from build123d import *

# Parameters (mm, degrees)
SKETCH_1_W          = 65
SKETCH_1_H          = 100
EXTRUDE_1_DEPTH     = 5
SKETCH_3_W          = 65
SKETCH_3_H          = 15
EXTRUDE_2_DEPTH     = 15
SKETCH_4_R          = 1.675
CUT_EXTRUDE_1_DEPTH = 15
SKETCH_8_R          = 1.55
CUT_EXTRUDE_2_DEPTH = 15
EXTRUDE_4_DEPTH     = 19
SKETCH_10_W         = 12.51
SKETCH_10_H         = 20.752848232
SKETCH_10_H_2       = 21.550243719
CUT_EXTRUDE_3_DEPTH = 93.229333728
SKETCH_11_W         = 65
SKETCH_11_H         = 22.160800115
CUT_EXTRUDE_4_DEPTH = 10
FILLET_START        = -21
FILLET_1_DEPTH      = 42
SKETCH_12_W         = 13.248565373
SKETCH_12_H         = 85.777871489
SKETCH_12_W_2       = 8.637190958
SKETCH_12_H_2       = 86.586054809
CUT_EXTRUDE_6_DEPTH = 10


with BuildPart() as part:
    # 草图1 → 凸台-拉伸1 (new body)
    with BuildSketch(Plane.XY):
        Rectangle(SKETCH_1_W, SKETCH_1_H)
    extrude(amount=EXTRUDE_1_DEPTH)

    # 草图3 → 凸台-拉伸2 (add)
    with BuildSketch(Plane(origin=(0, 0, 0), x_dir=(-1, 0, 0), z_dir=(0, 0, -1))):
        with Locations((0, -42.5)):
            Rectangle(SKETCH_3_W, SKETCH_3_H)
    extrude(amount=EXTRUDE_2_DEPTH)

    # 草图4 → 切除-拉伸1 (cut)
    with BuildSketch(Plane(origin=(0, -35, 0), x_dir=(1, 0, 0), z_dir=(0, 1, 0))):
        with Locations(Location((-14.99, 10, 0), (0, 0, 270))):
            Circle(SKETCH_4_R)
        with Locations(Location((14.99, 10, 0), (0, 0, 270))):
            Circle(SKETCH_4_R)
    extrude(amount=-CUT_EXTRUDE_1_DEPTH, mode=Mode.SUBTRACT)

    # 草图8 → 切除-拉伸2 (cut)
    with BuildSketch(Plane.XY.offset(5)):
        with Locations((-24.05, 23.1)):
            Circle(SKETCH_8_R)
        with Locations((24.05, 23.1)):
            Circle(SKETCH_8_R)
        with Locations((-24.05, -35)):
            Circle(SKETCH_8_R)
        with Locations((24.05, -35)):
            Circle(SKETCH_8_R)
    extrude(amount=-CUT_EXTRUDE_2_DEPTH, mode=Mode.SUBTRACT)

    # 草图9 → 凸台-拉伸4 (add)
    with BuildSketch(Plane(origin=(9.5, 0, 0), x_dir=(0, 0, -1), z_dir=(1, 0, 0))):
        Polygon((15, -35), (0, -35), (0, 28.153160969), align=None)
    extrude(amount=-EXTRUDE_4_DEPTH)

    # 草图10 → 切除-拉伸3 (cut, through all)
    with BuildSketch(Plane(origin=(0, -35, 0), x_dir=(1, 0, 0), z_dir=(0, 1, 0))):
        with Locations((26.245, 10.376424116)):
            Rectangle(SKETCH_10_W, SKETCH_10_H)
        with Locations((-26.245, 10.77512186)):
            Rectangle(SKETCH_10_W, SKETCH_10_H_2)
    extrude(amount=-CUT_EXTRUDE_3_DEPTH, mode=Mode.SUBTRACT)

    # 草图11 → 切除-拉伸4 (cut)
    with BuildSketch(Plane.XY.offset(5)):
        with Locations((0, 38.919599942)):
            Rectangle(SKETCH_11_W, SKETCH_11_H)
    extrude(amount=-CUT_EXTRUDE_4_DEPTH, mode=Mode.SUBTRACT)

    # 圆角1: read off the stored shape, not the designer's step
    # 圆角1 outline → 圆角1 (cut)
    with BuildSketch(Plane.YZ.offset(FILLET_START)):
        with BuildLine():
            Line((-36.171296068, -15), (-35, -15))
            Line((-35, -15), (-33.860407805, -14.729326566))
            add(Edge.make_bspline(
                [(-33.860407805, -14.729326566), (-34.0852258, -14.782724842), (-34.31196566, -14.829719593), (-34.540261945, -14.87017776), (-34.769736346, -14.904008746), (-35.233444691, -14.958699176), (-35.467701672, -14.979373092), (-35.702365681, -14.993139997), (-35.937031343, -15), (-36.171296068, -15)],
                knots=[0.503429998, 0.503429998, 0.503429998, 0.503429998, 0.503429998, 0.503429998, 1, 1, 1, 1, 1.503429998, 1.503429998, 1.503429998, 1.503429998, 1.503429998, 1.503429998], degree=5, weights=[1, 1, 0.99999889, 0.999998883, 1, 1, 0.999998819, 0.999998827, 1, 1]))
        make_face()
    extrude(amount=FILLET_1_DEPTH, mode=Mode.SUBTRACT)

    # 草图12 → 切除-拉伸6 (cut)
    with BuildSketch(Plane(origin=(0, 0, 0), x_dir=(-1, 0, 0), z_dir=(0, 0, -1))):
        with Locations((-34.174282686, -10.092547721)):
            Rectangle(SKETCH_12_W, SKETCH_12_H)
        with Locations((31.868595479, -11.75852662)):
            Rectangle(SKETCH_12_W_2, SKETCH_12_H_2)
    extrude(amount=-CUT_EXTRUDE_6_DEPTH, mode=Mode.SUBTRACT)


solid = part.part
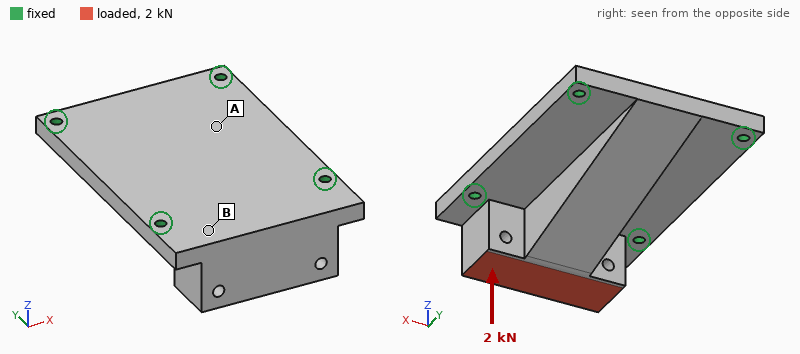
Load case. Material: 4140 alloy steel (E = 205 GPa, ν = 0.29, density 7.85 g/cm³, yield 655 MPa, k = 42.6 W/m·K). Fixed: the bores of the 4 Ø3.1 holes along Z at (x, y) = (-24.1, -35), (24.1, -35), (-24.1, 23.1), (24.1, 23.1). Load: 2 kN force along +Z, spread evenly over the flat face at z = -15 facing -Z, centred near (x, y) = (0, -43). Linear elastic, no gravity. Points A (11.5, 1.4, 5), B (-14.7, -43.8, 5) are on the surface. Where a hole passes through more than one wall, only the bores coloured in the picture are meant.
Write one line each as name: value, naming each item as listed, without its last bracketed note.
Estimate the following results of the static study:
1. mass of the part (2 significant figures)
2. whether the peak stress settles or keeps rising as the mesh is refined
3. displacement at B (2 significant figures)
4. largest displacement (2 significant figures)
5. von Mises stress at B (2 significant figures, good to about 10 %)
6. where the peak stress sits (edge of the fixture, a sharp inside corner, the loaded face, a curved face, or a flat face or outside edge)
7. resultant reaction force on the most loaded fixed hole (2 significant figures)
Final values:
mass of the part: 310 g
whether the peak stress settles or keeps rising as the mesh is refined: keeps rising
displacement at B: 5.6 µm
largest displacement: 8.7 µm
von Mises stress at B: 12 MPa
where the peak stress sits: edge of the fixture
resultant reaction force on the most loaded fixed hole: 1.2 kN
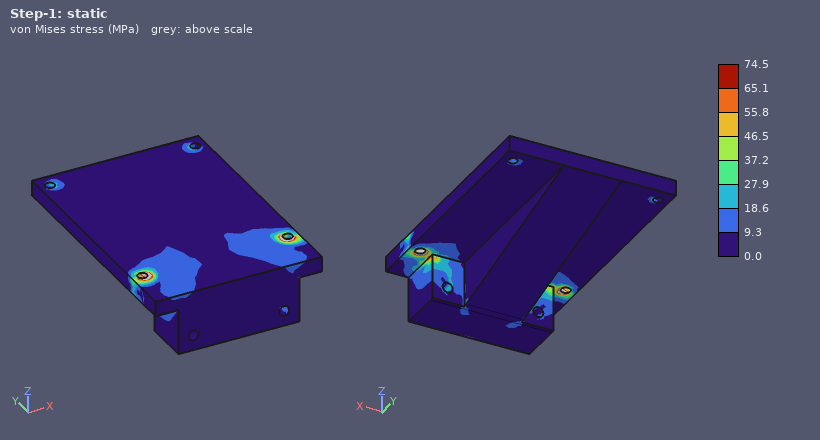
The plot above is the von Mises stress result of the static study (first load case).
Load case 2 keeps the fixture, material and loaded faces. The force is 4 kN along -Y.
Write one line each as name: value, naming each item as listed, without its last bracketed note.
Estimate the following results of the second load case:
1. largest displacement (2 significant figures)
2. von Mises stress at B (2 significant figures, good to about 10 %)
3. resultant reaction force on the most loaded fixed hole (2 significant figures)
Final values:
largest displacement: 21 µm
von Mises stress at B: 16 MPa
resultant reaction force on the most loaded fixed hole: 1.3 kN
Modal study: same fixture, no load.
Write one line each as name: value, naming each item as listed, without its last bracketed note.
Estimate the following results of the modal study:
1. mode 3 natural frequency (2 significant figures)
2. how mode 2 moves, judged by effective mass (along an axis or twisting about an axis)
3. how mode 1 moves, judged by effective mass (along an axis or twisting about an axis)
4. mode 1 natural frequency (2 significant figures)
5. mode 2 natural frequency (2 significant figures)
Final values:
mode 3 natural frequency: 11 kHz
how mode 2 moves, judged by effective mass: along Z
how mode 1 moves, judged by effective mass: along Z
mode 1 natural frequency: 5900 Hz
mode 2 natural frequency: 8300 Hz
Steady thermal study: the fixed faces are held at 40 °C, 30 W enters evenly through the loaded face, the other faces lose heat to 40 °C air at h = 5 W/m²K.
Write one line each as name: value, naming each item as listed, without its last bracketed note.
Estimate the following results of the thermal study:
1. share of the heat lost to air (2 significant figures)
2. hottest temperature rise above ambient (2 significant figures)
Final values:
share of the heat lost to air: 4.0 %
hottest temperature rise above ambient: 49 K
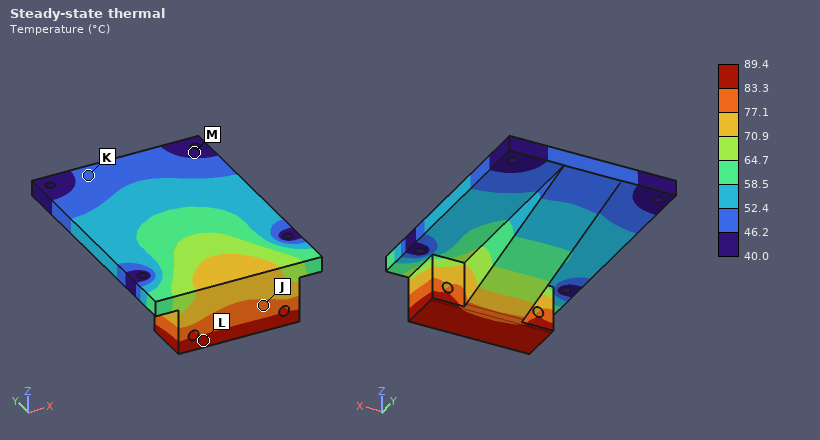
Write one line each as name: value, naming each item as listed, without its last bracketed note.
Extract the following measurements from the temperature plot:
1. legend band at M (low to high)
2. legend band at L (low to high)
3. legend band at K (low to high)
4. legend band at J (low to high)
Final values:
legend band at M: 40.0 to 46.2 °C
legend band at L: 83.3 to 89.4 °C
legend band at K: 46.2 to 52.4 °C
legend band at J: 77.1 to 83.3 °C
